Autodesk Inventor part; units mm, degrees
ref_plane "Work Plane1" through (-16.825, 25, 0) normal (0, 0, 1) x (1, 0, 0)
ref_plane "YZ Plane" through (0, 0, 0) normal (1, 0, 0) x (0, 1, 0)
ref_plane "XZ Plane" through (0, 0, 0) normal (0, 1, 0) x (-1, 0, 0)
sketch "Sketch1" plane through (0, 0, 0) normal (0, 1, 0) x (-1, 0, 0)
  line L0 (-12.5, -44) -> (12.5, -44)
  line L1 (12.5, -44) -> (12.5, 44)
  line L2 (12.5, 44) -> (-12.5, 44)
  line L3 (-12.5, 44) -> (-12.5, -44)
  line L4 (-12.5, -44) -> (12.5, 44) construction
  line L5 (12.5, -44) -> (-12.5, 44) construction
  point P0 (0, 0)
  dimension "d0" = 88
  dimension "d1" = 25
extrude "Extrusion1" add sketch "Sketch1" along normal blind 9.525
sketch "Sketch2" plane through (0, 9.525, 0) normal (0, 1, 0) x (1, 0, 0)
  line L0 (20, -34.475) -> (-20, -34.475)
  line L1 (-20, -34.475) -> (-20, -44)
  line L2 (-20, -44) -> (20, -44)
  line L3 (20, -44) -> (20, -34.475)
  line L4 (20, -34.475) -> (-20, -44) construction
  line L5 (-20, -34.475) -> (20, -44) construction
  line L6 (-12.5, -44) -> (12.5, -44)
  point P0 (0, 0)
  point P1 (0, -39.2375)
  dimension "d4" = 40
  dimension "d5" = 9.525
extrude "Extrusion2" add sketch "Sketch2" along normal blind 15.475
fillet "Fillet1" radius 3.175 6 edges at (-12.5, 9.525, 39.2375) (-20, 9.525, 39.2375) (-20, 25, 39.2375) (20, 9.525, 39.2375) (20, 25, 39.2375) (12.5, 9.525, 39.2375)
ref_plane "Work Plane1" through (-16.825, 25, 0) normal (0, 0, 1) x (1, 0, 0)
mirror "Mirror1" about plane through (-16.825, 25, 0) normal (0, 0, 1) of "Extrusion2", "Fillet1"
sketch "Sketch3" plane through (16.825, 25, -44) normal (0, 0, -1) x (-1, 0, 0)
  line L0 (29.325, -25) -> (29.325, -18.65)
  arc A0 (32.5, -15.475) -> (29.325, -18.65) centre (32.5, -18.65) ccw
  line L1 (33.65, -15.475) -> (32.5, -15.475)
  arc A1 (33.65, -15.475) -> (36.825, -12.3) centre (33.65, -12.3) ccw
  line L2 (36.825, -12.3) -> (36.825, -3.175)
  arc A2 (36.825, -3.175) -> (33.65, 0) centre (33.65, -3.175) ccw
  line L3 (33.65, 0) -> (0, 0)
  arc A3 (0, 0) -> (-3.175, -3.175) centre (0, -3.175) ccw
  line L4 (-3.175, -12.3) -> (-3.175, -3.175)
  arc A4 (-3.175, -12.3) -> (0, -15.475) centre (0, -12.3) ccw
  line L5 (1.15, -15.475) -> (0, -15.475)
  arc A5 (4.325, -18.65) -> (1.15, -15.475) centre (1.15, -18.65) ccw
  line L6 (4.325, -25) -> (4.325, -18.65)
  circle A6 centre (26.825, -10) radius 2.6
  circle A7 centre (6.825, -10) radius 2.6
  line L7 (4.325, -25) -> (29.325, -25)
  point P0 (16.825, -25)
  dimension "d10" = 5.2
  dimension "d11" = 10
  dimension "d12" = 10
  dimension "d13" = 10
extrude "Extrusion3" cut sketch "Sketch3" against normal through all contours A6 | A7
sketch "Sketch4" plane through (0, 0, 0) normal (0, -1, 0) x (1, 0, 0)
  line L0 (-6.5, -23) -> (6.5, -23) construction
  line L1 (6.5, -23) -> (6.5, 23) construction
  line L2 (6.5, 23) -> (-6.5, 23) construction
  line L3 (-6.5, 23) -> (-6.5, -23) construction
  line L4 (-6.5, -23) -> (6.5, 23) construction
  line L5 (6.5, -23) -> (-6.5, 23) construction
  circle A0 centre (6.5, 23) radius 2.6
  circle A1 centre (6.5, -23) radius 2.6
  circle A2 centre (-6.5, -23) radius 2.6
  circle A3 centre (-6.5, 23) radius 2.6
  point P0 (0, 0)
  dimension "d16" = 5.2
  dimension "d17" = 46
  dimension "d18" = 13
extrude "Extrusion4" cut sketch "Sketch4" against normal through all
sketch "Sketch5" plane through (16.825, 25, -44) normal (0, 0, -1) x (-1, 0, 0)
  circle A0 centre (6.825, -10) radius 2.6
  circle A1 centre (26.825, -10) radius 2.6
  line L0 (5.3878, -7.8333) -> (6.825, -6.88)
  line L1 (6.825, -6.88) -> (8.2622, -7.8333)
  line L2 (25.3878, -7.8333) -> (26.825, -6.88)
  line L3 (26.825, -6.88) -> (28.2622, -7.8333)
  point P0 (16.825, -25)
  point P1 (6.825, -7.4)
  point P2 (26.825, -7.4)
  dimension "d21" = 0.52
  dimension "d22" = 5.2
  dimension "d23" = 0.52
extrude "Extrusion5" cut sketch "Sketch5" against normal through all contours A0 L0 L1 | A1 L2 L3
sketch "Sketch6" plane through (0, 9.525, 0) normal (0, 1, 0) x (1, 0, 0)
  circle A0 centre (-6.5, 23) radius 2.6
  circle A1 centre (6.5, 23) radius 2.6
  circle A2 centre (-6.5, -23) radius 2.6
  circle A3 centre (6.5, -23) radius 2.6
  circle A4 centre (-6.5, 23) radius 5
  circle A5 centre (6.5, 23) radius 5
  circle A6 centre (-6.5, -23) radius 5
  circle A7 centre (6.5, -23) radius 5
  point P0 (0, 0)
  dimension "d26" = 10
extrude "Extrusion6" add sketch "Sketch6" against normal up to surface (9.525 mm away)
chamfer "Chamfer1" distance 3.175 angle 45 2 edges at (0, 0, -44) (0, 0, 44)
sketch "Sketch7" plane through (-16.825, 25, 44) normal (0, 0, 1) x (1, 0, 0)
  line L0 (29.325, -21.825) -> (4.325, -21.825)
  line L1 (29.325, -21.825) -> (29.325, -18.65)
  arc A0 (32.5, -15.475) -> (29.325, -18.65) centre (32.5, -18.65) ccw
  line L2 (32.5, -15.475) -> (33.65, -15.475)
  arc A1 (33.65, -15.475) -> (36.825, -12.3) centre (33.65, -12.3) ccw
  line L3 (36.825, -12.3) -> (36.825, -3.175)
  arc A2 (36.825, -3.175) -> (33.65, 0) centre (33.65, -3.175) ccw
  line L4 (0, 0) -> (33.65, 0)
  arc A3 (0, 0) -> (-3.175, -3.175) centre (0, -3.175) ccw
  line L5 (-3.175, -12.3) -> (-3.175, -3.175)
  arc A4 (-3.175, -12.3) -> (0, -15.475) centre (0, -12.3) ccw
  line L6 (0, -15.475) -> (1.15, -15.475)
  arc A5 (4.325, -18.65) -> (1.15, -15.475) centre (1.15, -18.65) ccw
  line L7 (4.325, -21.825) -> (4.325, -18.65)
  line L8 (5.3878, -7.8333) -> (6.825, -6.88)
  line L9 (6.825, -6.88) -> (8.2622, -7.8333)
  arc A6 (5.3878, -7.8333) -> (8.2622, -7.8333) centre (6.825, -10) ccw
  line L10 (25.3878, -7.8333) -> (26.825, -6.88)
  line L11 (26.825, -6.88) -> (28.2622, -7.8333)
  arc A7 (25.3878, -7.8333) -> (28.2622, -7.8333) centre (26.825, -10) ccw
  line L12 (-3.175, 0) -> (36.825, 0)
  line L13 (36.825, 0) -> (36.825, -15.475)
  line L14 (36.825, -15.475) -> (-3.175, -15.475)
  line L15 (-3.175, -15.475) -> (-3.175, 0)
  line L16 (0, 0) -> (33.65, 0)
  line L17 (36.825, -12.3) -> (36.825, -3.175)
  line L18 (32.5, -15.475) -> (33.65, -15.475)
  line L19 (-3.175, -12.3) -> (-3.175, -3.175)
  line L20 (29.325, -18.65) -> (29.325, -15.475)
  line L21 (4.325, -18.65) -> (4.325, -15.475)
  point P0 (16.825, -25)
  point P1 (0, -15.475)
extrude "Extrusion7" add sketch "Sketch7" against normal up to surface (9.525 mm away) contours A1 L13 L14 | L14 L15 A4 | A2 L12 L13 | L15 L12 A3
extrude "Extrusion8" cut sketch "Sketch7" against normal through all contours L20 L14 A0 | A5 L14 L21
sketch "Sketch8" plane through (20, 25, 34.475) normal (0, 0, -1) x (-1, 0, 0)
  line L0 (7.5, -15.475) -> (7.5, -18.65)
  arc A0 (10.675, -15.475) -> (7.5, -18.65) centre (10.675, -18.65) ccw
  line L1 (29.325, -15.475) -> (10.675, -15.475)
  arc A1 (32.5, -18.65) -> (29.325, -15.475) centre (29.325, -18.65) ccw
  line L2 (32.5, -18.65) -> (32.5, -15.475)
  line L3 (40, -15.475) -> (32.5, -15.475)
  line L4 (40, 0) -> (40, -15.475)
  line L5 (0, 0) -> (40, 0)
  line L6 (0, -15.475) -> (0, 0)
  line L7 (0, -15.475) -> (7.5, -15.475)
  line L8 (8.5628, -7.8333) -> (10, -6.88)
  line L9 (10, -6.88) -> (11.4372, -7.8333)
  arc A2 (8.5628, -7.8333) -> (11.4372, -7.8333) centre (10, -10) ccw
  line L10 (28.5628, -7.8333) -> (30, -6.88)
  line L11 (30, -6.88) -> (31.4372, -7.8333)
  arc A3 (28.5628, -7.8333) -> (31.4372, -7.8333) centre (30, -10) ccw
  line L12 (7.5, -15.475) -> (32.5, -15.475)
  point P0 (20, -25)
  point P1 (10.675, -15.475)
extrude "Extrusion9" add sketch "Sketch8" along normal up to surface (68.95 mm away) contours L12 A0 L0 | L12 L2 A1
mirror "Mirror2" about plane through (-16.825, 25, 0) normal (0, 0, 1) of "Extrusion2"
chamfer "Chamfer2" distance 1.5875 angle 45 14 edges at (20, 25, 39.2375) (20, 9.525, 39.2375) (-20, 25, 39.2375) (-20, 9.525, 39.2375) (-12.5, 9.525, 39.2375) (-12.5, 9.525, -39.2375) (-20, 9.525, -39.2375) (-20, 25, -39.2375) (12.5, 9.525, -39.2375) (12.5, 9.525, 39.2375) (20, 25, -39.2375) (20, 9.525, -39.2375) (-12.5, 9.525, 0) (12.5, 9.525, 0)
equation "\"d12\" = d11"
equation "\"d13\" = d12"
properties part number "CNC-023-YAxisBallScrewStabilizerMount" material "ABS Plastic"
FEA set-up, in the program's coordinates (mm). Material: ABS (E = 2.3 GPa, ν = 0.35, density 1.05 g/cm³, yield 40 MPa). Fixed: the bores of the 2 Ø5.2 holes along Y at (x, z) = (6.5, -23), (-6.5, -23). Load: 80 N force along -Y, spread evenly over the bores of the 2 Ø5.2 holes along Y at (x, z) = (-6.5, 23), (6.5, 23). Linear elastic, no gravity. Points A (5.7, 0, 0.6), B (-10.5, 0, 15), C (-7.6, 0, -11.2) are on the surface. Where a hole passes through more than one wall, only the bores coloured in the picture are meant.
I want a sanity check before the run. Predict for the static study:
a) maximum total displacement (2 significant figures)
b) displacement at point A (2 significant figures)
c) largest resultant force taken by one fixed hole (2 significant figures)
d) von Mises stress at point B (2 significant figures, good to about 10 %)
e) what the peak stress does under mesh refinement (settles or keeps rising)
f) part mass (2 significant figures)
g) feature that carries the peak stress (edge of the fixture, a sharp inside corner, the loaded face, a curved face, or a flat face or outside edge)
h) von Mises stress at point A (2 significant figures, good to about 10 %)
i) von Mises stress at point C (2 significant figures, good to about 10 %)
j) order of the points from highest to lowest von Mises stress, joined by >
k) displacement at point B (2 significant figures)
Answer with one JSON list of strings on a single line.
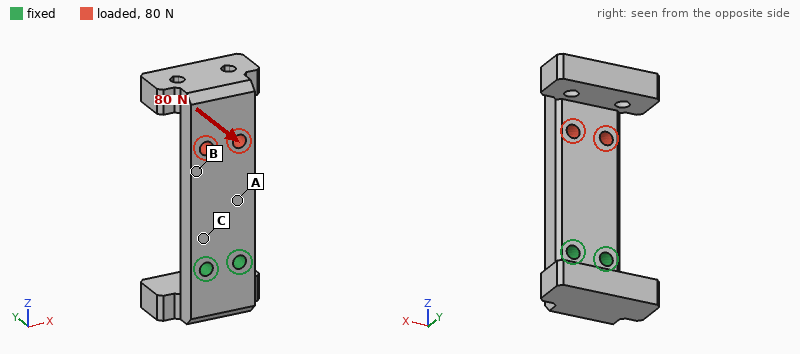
["1.1 mm", "0.21 mm", "40 N", "1.8 MPa", "keeps rising", "33 g", "edge of the fixture", "4.8 MPa", "7.3 MPa", "C > A > B", "0.45 mm"]
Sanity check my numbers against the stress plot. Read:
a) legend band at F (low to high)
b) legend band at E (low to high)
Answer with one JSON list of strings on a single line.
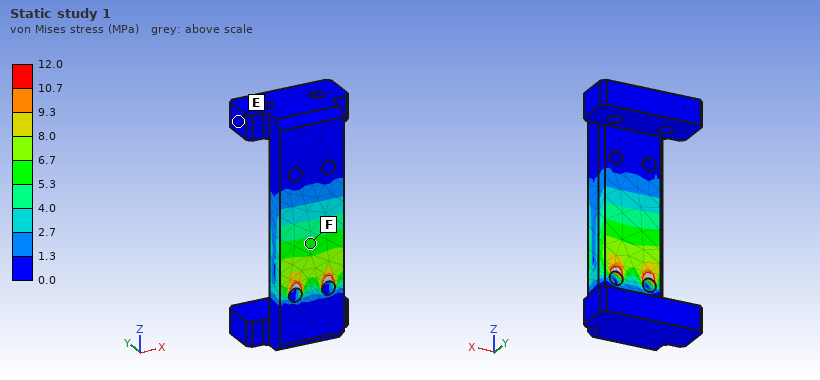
["5.3 to 6.7 MPa", "0.0 to 1.3 MPa"]
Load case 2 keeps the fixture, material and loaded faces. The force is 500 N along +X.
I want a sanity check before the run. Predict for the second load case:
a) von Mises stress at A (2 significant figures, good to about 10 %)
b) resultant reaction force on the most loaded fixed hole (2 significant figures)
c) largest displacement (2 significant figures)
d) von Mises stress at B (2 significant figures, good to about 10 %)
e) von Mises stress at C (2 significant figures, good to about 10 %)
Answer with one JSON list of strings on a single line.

["7.0 MPa", "1.4 kN", "1.2 mm", "3.7 MPa", "12 MPa"]
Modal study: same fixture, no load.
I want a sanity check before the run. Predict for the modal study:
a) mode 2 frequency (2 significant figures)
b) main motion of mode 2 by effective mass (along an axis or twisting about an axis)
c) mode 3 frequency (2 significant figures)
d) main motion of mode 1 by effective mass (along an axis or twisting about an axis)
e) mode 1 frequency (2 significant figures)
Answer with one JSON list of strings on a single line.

["730 Hz", "along X", "1200 Hz", "along Y", "350 Hz"]
